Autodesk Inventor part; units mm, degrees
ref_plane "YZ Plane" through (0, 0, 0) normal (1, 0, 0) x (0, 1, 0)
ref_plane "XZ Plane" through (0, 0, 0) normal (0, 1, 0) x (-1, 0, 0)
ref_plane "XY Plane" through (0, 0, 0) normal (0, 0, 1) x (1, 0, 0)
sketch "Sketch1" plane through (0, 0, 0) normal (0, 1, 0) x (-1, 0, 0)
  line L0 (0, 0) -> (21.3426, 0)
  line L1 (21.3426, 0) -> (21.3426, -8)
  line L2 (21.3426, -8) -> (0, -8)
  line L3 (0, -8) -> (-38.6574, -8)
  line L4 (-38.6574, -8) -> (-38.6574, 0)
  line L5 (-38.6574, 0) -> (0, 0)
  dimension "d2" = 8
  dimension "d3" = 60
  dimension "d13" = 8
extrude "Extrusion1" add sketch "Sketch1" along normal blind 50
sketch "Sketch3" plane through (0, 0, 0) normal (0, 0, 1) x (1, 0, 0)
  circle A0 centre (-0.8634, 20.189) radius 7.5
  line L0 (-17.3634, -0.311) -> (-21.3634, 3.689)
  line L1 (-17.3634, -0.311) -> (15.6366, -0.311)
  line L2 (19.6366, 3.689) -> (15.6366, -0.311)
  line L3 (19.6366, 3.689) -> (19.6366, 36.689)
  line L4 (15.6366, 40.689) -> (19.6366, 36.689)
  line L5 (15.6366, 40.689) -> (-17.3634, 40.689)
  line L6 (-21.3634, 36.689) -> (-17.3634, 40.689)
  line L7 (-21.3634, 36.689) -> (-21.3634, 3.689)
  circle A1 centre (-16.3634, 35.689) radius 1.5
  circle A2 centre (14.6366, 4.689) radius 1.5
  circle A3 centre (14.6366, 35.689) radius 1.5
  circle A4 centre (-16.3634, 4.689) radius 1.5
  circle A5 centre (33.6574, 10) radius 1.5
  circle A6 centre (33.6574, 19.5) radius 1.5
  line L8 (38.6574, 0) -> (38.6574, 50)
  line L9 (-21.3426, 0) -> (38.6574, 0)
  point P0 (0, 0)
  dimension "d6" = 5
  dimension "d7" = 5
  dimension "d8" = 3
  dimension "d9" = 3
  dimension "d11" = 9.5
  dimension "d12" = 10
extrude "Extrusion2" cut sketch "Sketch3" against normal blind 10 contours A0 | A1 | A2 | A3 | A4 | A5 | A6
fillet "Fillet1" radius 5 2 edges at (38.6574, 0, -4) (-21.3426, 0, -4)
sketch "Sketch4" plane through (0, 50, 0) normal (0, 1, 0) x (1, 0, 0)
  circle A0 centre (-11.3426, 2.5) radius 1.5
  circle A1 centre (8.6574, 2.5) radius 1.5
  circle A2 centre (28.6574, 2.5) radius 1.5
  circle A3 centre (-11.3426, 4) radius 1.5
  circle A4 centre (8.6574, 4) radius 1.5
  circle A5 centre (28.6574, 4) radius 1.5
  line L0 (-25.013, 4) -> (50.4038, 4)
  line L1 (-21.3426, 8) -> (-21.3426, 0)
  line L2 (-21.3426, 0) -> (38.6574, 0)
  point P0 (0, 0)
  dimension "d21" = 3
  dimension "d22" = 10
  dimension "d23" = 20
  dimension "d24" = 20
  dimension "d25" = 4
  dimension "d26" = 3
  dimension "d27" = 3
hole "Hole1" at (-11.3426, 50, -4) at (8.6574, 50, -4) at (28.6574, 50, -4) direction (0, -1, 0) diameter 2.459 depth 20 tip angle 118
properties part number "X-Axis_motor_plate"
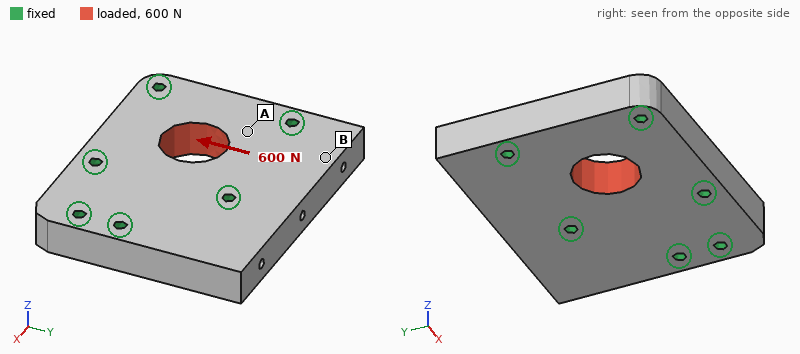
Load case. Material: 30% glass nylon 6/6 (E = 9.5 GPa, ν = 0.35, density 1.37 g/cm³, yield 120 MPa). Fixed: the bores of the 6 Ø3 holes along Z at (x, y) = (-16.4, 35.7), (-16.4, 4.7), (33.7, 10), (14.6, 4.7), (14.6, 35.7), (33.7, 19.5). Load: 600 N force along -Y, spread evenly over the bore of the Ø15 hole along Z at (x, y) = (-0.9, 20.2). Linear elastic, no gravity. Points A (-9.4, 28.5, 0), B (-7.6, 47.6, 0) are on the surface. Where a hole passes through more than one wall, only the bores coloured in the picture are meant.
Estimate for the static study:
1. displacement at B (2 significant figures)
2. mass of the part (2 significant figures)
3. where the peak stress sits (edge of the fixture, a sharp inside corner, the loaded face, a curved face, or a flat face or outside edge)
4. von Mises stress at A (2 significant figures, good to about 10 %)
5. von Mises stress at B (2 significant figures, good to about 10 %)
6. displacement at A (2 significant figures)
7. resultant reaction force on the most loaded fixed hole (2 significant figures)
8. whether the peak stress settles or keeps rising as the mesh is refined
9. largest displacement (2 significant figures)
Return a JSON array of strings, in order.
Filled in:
["1.9 µm", "30 g", "edge of the fixture", "1.7 MPa", "0.65 MPa", "2.3 µm", "160 N", "keeps rising", "4.9 µm"]
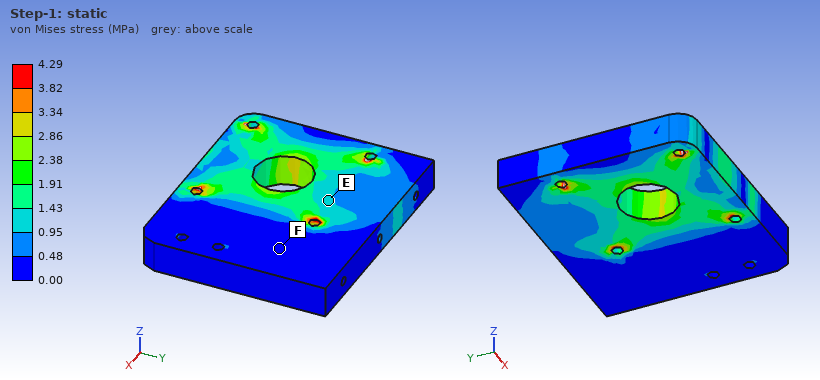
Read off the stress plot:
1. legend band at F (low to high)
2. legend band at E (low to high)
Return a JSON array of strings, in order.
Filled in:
["0.00 to 0.48 MPa", "0.95 to 1.43 MPa"]
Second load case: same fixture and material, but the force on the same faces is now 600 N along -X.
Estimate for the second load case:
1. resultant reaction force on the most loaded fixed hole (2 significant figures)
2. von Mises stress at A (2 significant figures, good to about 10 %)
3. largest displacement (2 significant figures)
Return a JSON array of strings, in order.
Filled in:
["140 N", "1.8 MPa", "5.0 µm"]
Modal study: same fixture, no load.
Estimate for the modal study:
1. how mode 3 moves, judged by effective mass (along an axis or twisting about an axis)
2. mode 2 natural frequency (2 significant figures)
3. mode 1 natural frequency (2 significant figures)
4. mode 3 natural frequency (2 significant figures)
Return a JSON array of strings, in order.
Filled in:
["along Z", "10 kHz", "6800 Hz", "13 kHz"]
